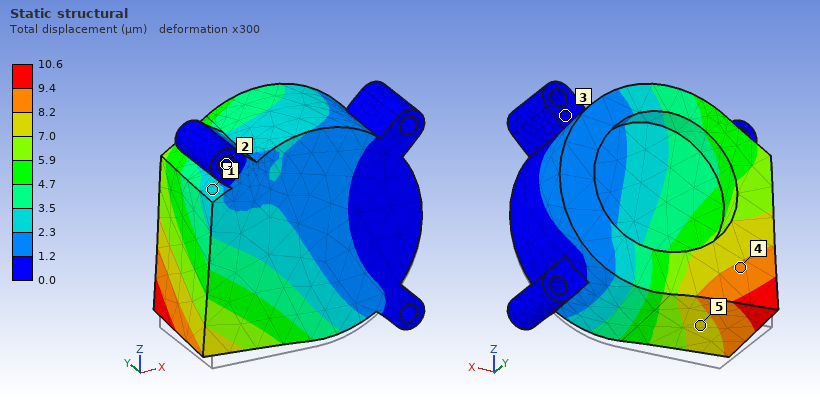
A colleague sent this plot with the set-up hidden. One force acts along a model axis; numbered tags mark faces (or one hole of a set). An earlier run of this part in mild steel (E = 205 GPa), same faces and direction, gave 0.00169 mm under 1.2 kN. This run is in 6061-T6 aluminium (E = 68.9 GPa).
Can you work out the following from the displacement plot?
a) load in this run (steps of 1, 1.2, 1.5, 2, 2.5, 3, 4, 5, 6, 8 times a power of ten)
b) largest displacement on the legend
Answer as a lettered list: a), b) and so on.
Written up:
a) 2.5 kN
b) 10.6 µm
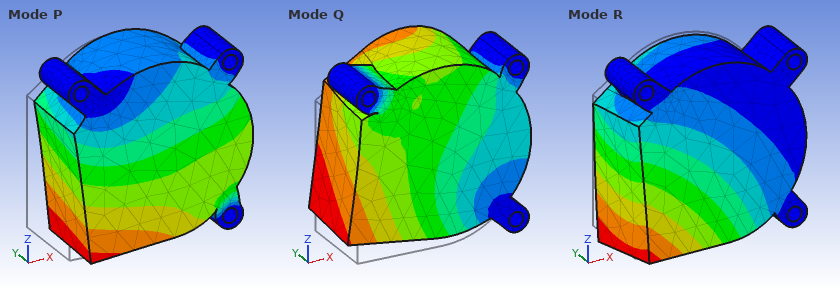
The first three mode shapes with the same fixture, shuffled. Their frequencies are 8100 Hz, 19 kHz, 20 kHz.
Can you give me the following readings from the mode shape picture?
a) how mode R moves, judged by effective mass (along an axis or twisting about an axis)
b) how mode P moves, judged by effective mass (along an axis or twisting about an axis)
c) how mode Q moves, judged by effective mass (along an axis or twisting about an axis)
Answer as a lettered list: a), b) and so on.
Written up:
a) along Y
b) along X
c) along Z
